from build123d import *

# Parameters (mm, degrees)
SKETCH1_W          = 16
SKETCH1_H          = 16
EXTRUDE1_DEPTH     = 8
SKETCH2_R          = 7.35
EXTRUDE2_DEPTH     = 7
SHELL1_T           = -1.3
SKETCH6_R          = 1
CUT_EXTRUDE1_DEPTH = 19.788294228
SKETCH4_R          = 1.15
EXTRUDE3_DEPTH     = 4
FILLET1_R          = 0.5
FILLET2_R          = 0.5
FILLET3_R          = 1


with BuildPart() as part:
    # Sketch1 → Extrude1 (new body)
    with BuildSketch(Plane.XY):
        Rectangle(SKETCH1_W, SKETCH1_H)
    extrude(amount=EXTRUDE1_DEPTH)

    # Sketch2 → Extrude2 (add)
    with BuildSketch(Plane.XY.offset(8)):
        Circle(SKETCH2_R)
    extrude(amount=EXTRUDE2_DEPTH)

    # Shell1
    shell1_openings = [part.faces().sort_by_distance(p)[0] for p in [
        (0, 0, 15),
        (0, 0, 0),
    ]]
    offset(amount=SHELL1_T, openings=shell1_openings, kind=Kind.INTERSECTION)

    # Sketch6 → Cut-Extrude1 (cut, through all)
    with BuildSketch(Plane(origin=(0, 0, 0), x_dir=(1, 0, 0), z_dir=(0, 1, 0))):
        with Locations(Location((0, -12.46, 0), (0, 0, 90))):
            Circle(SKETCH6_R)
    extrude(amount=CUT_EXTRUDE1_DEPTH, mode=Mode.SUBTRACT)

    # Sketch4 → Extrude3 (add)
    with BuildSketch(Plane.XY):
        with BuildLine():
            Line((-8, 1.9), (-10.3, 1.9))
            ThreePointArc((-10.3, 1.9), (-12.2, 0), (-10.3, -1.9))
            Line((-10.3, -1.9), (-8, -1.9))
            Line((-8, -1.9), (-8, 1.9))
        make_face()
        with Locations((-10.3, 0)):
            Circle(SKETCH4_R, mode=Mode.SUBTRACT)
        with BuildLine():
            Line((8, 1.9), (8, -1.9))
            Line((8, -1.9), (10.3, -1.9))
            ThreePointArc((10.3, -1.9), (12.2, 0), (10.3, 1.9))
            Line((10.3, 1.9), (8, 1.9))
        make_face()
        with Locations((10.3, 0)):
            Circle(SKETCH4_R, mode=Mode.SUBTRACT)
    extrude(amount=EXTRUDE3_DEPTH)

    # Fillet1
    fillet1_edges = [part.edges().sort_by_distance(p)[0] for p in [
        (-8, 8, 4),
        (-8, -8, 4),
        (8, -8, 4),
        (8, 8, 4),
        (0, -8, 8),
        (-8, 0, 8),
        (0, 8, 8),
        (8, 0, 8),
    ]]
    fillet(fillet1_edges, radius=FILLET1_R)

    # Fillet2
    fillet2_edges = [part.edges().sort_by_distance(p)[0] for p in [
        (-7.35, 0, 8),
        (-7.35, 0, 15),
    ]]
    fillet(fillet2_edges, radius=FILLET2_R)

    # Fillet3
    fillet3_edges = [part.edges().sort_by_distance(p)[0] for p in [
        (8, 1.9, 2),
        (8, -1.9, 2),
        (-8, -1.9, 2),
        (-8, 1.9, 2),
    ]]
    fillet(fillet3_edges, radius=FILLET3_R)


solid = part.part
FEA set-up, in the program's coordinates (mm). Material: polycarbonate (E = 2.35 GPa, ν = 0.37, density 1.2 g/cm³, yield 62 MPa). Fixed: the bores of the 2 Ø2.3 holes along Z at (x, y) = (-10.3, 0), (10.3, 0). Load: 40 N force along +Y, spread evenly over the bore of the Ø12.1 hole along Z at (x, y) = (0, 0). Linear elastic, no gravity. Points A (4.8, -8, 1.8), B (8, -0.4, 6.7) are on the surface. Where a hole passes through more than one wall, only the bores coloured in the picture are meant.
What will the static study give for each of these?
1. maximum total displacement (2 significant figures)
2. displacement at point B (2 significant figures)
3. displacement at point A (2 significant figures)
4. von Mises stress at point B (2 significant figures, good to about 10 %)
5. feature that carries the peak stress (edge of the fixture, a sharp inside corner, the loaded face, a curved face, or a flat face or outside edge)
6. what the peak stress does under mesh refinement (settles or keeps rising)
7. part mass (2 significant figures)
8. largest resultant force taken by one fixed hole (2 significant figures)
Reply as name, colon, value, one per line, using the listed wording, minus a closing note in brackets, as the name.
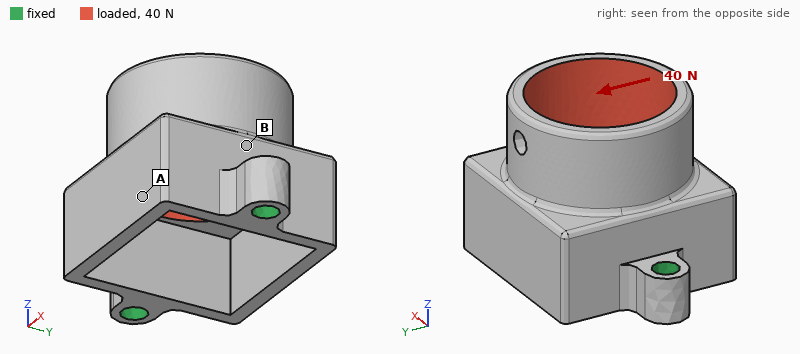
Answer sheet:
maximum total displacement: 0.21 mm
displacement at point B: 0.067 mm
displacement at point A: 0.11 mm
von Mises stress at point B: 4.2 MPa
feature that carries the peak stress: edge of the fixture
what the peak stress does under mesh refinement: keeps rising
part mass: 1.4 g
largest resultant force taken by one fixed hole: 20 N
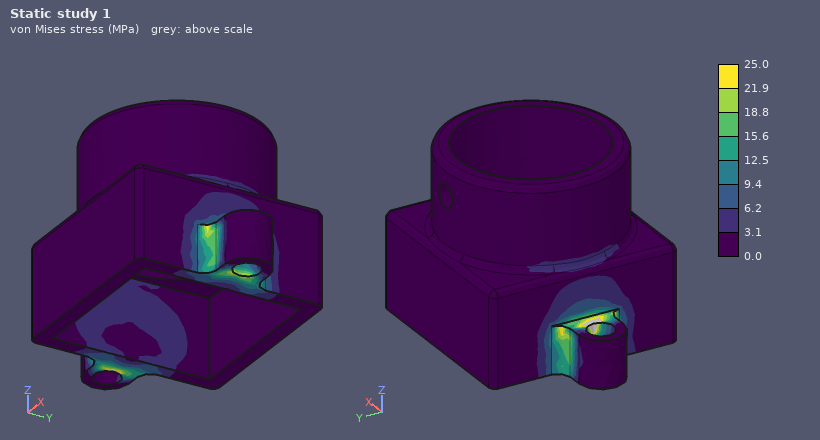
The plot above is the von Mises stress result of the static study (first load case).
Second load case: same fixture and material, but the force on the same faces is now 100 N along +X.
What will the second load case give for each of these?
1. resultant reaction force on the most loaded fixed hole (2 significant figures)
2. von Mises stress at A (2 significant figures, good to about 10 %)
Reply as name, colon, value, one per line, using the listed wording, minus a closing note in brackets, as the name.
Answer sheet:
resultant reaction force on the most loaded fixed hole: 66 N
von Mises stress at A: 4.0 MPa
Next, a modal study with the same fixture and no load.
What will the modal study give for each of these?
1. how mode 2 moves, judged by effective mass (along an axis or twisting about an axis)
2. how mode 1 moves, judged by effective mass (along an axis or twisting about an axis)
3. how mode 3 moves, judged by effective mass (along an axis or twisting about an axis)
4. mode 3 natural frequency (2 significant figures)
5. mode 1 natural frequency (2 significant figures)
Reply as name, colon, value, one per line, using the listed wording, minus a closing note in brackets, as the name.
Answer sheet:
how mode 2 moves, judged by effective mass: along X
how mode 1 moves, judged by effective mass: along Y
how mode 3 moves, judged by effective mass: twisting about Z
mode 3 natural frequency: 5000 Hz
mode 1 natural frequency: 2700 Hz
